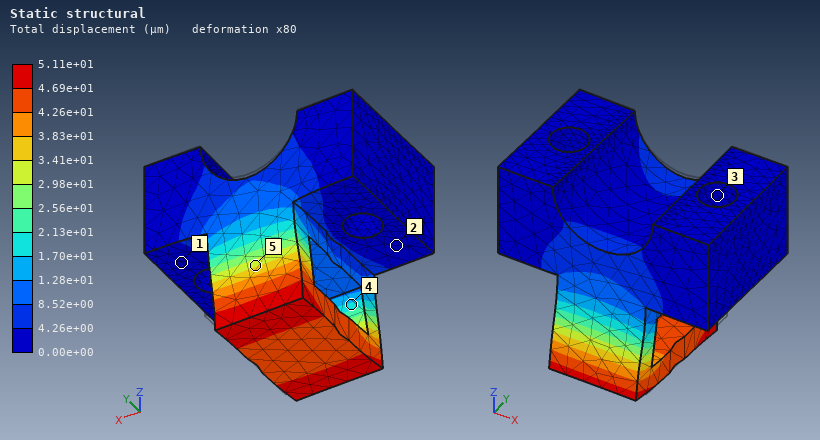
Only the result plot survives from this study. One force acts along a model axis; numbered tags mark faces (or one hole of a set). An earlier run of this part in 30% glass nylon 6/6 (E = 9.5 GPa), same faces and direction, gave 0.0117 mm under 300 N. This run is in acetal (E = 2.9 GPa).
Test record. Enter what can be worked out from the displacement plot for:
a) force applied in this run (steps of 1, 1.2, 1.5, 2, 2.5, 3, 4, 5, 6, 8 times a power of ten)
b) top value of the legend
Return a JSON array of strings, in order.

["400 N", "5.11e+01 µm"]
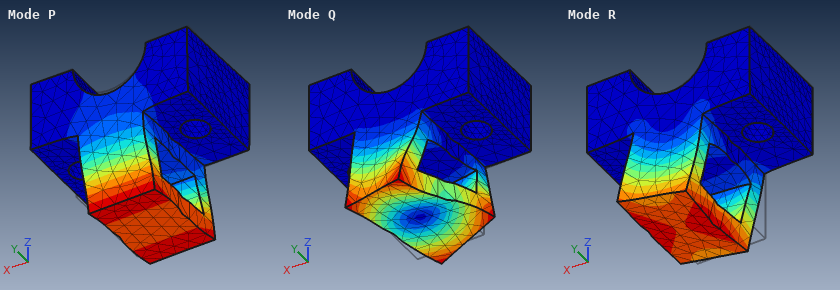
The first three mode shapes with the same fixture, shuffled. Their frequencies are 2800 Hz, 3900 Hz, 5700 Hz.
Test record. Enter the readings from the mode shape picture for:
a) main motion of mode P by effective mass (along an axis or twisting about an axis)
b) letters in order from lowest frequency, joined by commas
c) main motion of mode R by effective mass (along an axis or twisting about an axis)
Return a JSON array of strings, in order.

["along Y", "P, R, Q", "along X"]
